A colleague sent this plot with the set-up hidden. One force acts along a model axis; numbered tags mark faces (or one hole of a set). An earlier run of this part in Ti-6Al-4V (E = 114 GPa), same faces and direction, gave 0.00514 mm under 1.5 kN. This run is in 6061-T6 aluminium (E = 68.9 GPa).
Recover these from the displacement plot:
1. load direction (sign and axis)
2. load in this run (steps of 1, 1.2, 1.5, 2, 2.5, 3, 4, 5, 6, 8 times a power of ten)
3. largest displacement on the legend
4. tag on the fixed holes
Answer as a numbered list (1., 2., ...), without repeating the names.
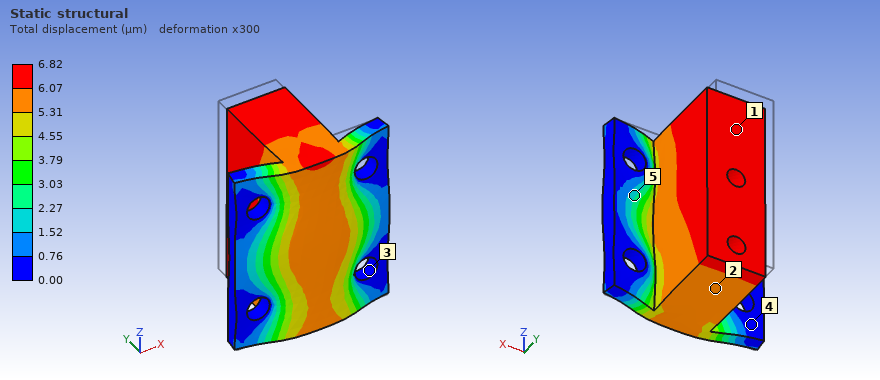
1. -Y
2. 1.2 kN
3. 6.82 µm
4. 3
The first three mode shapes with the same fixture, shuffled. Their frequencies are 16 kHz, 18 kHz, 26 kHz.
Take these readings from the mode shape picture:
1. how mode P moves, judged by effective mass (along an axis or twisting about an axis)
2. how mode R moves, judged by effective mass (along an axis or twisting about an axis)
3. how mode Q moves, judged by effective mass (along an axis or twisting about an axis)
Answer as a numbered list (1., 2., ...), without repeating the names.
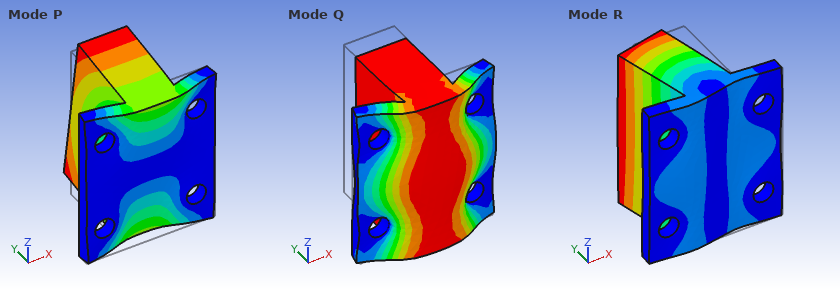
1. along Z
2. along X
3. along Y
